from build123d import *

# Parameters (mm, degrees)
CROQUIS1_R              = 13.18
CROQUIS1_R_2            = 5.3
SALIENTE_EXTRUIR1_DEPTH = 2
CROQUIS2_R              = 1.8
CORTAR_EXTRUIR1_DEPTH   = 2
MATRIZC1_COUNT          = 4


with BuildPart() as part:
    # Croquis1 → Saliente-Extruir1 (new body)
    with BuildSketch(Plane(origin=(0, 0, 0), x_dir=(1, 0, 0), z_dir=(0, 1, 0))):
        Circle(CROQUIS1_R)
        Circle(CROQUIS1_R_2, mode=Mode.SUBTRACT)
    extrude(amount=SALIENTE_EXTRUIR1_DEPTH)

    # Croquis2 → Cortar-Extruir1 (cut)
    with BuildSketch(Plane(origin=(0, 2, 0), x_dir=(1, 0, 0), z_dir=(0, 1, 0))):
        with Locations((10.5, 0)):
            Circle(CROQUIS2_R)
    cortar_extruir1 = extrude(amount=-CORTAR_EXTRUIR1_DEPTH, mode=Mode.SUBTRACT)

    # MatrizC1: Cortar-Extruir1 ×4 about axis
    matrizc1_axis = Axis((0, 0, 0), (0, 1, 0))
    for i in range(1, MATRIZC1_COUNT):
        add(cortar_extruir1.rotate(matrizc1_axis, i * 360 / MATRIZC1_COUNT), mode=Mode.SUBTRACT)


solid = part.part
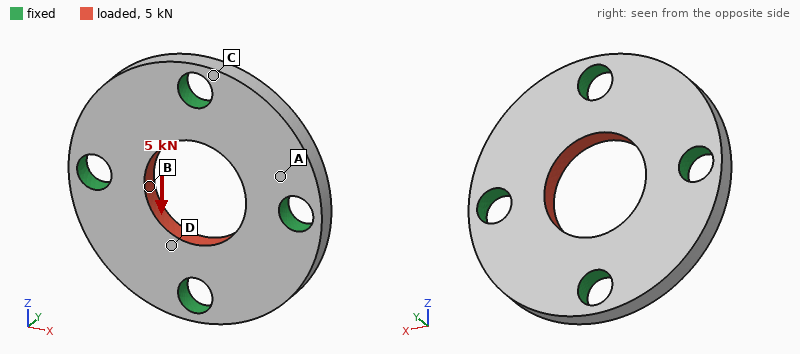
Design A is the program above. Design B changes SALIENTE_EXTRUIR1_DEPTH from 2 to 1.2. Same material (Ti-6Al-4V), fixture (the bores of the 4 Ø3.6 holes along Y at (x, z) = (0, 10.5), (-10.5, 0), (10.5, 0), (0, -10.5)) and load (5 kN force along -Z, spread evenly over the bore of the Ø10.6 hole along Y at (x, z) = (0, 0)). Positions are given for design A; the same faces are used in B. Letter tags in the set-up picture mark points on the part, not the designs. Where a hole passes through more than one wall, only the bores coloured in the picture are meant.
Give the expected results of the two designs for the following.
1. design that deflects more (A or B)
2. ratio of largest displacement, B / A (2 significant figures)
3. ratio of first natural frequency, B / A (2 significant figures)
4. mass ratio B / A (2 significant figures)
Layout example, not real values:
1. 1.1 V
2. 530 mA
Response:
1. B
2. 1.7
3. 0.67
4. 0.60
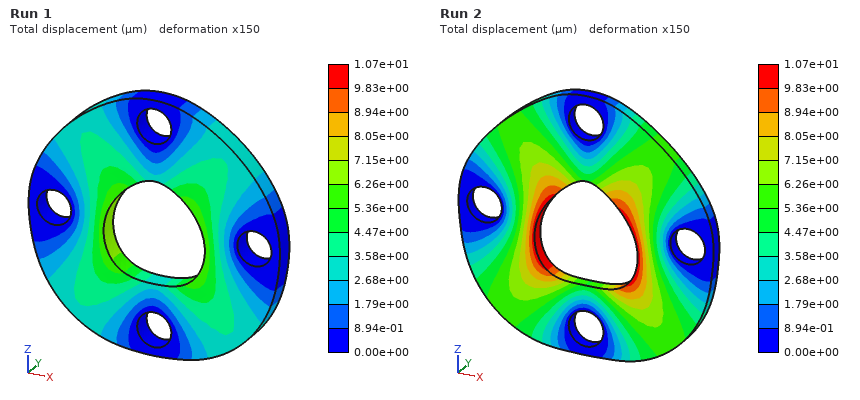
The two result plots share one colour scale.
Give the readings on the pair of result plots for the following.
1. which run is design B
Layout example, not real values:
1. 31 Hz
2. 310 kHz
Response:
1. Run 2
